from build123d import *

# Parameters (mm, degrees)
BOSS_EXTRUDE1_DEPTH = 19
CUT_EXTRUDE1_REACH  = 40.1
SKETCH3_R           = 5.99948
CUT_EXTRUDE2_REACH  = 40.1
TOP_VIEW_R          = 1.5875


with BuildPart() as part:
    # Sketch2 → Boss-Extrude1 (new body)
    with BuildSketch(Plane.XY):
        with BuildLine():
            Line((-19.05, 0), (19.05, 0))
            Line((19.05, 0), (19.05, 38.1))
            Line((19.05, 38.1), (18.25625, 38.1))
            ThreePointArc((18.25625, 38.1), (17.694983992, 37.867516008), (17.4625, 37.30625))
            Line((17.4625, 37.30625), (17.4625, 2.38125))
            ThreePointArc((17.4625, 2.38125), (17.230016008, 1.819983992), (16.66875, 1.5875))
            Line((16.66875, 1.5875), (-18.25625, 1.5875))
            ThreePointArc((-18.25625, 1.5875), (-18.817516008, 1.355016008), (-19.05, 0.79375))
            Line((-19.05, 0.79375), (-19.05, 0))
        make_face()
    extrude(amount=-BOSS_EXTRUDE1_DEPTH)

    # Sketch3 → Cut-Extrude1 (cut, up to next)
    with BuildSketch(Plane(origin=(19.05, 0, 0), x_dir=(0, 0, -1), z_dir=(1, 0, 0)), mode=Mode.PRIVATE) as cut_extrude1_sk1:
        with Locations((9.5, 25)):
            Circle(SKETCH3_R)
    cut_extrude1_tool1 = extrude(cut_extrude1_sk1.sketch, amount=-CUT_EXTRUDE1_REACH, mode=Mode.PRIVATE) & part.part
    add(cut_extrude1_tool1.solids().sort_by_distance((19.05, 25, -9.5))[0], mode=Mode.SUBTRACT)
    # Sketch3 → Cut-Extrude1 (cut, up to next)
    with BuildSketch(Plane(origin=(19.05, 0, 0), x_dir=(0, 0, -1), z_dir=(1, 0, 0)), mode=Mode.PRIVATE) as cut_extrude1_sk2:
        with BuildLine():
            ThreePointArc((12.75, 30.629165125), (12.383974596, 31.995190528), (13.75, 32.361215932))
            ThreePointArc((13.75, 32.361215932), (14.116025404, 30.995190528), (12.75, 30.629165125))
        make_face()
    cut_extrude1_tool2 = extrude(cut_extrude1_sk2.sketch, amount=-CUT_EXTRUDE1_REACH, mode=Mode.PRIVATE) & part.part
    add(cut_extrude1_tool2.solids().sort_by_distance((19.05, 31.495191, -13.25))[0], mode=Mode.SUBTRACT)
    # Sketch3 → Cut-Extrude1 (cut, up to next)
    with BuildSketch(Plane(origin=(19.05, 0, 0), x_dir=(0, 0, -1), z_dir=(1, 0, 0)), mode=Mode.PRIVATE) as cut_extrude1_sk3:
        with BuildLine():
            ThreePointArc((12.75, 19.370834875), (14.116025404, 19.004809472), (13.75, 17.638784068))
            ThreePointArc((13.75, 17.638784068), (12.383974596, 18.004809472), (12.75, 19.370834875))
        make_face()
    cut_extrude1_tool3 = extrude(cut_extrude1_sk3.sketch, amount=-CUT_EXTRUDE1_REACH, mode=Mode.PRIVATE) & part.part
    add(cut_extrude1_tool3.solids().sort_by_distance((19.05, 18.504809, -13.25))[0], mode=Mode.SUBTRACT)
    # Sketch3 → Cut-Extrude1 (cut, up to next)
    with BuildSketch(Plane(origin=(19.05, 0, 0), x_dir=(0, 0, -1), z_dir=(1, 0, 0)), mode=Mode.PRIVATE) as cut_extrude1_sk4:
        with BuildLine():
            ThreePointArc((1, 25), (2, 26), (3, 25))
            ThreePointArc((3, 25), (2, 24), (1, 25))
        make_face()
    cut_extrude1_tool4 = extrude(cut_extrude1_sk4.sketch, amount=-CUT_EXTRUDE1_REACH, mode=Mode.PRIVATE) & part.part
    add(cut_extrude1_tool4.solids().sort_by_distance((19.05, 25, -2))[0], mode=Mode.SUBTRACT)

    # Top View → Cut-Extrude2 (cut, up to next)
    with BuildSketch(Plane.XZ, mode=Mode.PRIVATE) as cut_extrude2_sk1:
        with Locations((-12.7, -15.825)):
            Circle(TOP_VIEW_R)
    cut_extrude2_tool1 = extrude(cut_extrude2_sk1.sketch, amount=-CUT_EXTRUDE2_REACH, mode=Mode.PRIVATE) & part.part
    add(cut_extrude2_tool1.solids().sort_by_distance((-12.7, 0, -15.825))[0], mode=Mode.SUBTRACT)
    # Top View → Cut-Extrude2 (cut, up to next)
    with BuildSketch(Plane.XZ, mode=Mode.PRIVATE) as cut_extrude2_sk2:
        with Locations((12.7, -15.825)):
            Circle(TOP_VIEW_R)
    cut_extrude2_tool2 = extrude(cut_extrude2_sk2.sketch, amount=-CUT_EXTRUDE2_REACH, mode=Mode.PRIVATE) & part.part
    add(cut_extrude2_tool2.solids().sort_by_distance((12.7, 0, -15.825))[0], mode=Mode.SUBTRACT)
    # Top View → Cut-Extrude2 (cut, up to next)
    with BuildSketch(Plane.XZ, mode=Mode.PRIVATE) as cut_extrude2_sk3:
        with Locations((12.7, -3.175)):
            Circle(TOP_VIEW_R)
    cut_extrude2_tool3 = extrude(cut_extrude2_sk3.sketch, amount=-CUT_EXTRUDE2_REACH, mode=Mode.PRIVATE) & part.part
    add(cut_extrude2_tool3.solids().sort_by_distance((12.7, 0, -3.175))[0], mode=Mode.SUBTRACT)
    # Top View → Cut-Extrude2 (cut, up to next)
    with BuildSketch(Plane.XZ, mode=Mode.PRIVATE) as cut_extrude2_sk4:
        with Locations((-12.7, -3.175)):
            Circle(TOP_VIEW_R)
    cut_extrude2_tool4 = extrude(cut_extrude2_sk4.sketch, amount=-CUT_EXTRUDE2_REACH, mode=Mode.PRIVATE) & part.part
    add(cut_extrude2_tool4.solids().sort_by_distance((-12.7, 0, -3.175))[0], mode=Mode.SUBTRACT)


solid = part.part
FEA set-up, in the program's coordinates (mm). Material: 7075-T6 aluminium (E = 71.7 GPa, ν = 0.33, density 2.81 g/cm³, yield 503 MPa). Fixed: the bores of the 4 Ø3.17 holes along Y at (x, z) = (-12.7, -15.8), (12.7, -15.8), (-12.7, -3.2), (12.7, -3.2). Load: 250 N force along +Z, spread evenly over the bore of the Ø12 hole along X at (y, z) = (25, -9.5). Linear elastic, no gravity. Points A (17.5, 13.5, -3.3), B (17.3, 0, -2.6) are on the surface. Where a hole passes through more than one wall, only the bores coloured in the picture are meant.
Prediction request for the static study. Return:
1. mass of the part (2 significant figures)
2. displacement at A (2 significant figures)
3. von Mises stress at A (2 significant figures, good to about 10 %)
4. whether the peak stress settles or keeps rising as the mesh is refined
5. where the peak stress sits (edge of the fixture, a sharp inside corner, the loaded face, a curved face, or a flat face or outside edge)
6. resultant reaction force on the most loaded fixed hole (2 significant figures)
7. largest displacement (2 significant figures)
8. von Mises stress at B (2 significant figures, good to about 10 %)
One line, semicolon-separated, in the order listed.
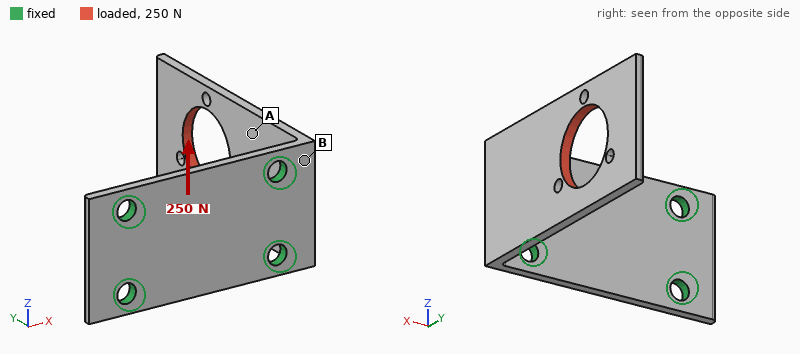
5.6 g; 0.12 mm; 31 MPa; keeps rising; edge of the fixture; 470 N; 0.34 mm; 120 MPa
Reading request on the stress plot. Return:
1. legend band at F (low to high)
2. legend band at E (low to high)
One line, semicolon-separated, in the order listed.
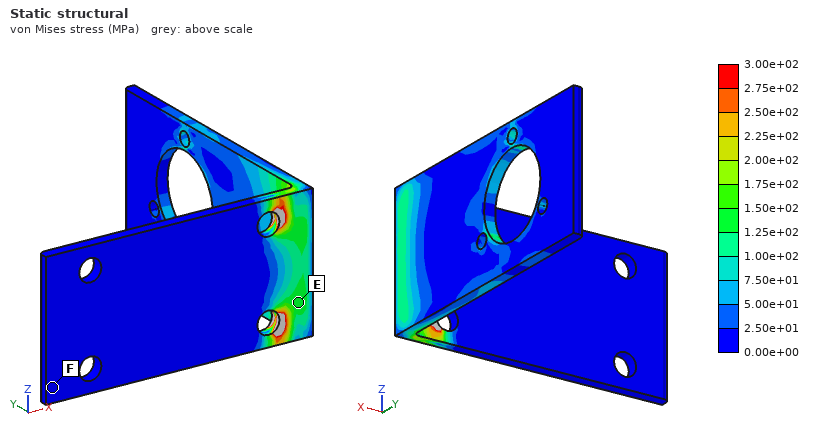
0.00e+00 to 2.50e+01 MPa; 1.25e+02 to 1.50e+02 MPa
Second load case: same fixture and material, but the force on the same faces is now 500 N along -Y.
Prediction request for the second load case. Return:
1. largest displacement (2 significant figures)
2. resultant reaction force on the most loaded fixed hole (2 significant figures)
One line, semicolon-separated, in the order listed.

0.43 mm; 250 N
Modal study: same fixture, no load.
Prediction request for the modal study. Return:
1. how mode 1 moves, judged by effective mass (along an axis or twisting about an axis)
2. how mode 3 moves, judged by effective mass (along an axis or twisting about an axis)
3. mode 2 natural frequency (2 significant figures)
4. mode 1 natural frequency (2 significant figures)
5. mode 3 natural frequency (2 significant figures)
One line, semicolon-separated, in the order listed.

along X; along Z; 3300 Hz; 880 Hz; 4100 Hz
